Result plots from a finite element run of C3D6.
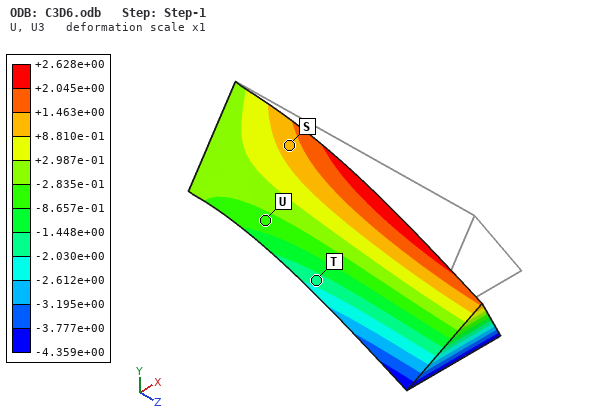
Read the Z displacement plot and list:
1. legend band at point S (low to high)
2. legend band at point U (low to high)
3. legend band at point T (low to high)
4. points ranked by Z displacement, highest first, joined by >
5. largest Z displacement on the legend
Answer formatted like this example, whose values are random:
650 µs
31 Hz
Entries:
+8.810e-01 to +1.463e+00
-8.657e-01 to -2.835e-01
-2.030e+00 to -1.448e+00
S > U > T
+2.628e+00
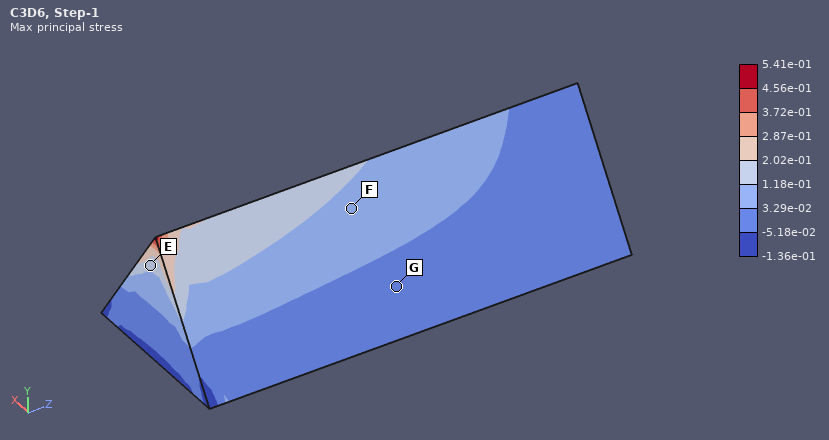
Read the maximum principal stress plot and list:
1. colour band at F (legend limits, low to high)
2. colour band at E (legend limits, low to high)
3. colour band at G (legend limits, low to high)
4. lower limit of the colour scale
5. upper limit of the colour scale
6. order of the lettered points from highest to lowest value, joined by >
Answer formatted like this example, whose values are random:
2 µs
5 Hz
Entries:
3.29e-02 to 1.18e-01
1.18e-01 to 2.02e-01
-5.18e-02 to 3.29e-02
-1.36e-01
5.41e-01
E > F > G
